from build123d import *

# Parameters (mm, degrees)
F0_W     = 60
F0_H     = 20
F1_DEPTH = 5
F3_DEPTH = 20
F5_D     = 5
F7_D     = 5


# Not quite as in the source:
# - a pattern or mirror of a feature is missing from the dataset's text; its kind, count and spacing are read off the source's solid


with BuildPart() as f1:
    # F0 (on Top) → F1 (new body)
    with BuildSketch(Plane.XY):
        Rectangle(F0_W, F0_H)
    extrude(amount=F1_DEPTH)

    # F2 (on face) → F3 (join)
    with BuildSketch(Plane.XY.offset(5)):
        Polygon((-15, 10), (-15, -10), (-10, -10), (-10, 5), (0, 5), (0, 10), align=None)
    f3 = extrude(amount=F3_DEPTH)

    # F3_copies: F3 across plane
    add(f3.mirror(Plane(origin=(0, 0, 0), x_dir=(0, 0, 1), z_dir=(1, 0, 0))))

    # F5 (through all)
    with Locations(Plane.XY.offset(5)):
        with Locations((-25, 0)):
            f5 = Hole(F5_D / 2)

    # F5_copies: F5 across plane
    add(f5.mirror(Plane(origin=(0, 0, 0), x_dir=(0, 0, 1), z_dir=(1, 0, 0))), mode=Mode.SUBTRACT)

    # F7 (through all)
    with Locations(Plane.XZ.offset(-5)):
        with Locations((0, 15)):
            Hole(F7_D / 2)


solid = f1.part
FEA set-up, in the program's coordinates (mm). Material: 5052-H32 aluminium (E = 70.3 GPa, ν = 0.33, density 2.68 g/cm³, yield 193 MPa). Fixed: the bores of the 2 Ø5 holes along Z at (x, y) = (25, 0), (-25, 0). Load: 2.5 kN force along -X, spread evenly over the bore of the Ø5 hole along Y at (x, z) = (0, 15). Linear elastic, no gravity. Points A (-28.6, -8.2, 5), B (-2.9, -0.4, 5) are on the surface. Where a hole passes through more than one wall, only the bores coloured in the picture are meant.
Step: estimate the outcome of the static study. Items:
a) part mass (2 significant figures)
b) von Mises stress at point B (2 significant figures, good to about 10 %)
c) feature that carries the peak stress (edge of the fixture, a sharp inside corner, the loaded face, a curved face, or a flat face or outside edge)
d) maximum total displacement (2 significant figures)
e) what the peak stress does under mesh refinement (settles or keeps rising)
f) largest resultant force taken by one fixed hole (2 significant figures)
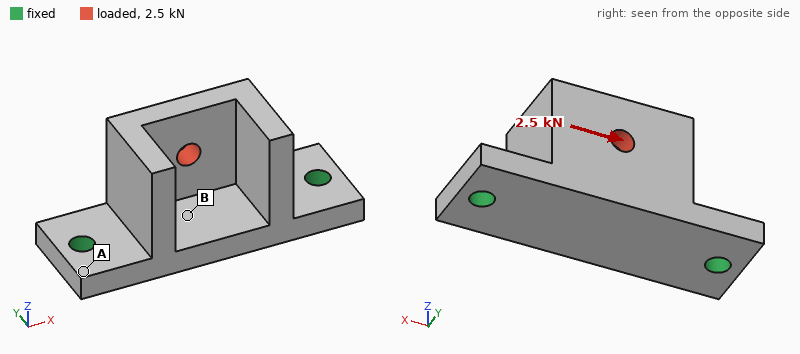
31 g
16 MPa
edge of the fixture
37 µm
keeps rising
1.5 kN
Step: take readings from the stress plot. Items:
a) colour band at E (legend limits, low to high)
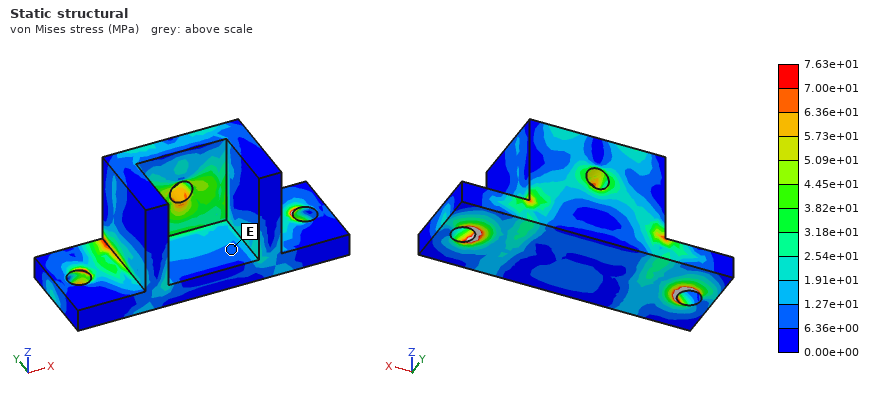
6.36e+00 to 1.27e+01 MPa
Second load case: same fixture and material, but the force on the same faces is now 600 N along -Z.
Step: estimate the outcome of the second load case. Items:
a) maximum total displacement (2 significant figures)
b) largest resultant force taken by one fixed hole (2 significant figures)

30 µm
330 N
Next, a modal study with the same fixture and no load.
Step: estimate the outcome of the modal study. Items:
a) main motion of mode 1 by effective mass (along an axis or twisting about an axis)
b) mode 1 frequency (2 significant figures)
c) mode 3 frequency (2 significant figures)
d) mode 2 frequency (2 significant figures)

along Y
5000 Hz
9900 Hz
9500 Hz
